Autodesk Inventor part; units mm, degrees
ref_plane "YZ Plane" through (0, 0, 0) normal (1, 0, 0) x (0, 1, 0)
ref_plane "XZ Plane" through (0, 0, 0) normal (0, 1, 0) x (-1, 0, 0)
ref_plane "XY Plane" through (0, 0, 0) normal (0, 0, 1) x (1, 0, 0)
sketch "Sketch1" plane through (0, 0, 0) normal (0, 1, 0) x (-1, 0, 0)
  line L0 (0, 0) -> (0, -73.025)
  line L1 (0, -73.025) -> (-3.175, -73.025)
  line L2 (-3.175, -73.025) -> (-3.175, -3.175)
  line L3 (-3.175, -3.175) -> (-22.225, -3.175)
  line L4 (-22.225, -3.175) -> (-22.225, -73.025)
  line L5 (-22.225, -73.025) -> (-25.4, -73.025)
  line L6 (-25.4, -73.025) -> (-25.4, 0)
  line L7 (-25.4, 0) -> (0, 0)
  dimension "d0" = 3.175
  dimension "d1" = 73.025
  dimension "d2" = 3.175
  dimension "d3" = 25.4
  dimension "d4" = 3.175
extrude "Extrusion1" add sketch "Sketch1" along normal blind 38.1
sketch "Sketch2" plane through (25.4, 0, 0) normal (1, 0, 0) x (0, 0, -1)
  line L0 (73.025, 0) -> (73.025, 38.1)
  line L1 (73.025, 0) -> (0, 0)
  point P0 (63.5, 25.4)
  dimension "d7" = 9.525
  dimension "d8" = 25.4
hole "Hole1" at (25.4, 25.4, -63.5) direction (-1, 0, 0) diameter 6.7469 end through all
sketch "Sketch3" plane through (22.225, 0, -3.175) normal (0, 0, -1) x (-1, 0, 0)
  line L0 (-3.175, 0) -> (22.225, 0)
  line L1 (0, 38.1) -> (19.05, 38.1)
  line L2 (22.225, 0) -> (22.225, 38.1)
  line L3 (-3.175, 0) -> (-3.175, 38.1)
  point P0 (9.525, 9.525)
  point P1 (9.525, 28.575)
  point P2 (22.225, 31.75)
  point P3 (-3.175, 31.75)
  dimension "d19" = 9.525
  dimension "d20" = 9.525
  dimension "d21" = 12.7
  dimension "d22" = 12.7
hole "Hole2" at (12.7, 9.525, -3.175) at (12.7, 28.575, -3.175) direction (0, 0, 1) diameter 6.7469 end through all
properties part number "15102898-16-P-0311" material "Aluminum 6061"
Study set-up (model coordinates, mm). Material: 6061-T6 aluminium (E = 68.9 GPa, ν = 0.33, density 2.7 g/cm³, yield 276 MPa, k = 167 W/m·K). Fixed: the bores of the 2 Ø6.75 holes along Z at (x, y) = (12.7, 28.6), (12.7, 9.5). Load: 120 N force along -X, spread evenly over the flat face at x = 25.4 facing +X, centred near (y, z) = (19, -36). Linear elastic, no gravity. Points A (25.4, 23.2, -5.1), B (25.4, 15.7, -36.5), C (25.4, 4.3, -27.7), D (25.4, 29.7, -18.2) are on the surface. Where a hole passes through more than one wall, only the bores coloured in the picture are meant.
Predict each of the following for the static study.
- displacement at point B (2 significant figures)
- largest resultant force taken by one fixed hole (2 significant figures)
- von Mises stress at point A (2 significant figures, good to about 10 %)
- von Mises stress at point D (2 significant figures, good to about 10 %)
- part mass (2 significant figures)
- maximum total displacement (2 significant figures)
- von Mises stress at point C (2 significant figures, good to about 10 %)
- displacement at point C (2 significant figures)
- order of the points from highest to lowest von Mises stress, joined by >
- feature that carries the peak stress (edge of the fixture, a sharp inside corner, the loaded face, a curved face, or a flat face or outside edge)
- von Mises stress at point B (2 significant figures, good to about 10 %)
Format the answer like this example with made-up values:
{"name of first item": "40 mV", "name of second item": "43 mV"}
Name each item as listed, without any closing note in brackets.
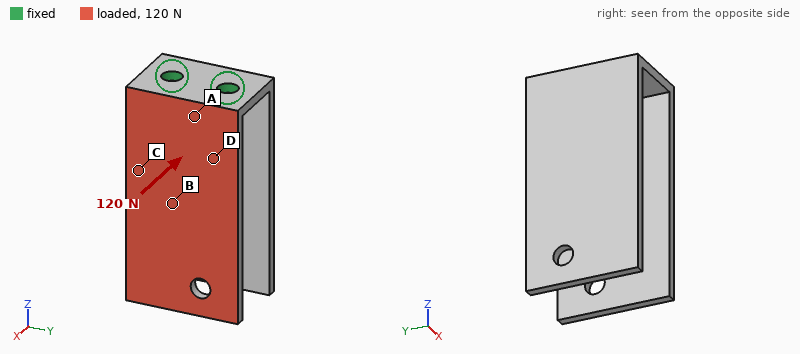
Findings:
{"displacement at point B": "0.40 mm", "largest resultant force taken by one fixed hole": "67 N", "von Mises stress at point A": "53 MPa", "von Mises stress at point D": "36 MPa", "part mass": "53 g", "maximum total displacement": "1.0 mm", "von Mises stress at point C": "26 MPa", "displacement at point C": "0.26 mm", "order of the points from highest to lowest von Mises stress, joined by >": "A > D > C > B", "feature that carries the peak stress": "a flat face or outside edge", "von Mises stress at point B": "16 MPa"}
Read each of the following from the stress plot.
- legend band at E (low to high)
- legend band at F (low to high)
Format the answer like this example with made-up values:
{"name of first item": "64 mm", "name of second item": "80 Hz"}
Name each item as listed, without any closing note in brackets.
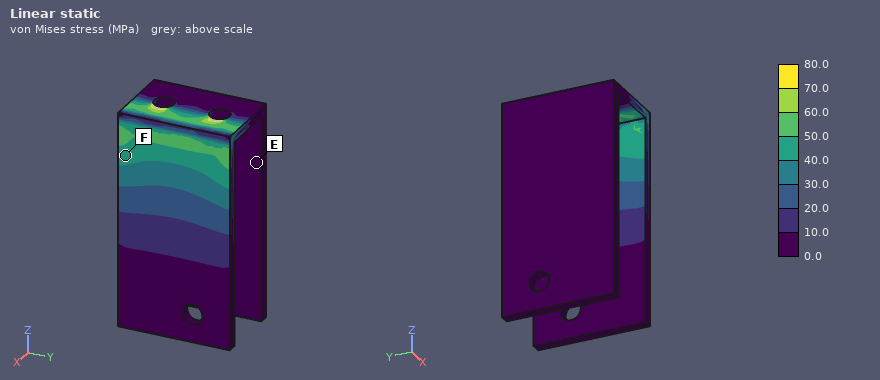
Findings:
{"legend band at E": "0.0 to 10.0 MPa", "legend band at F": "40.0 to 50.0 MPa"}
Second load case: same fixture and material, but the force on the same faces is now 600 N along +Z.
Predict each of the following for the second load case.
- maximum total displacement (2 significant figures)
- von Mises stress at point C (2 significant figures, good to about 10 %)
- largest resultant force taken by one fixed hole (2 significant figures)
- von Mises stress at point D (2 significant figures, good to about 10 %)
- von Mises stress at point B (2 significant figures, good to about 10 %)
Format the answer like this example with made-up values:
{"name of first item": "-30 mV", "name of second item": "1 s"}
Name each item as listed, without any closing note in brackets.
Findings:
{"maximum total displacement": "0.53 mm", "von Mises stress at point C": "12 MPa", "largest resultant force taken by one fixed hole": "300 N", "von Mises stress at point D": "14 MPa", "von Mises stress at point B": "9.5 MPa"}
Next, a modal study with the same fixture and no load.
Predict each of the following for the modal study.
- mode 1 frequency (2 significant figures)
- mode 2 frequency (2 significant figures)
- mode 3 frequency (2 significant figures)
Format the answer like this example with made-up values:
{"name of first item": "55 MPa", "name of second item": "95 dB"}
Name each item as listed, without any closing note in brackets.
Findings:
{"mode 1 frequency": "440 Hz", "mode 2 frequency": "440 Hz", "mode 3 frequency": "1600 Hz"}
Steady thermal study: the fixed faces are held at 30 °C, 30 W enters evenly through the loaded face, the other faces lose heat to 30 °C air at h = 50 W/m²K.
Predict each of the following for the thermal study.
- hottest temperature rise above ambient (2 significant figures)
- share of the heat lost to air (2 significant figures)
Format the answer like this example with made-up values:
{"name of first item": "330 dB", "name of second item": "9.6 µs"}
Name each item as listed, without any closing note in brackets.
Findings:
{"hottest temperature rise above ambient": "49 K", "share of the heat lost to air": "22 %"}
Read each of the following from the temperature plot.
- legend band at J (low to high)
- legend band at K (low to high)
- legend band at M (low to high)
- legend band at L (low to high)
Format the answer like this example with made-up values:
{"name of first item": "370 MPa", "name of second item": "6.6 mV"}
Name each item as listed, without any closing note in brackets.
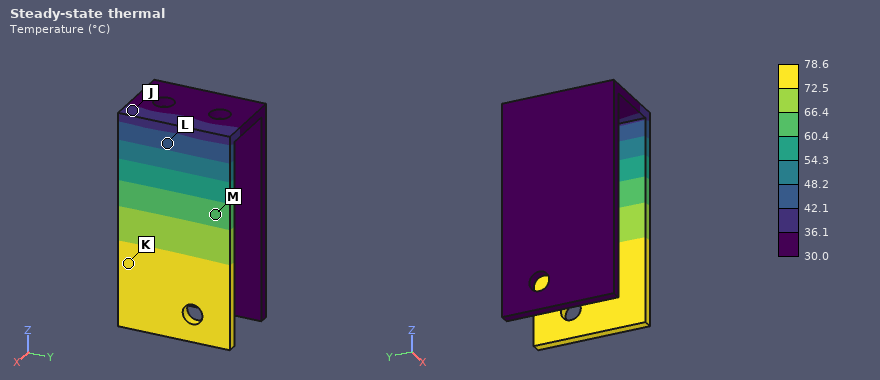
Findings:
{"legend band at J": "36.1 to 42.1 °C", "legend band at K": "72.5 to 78.6 °C", "legend band at M": "60.4 to 66.4 °C", "legend band at L": "42.1 to 48.2 °C"}
